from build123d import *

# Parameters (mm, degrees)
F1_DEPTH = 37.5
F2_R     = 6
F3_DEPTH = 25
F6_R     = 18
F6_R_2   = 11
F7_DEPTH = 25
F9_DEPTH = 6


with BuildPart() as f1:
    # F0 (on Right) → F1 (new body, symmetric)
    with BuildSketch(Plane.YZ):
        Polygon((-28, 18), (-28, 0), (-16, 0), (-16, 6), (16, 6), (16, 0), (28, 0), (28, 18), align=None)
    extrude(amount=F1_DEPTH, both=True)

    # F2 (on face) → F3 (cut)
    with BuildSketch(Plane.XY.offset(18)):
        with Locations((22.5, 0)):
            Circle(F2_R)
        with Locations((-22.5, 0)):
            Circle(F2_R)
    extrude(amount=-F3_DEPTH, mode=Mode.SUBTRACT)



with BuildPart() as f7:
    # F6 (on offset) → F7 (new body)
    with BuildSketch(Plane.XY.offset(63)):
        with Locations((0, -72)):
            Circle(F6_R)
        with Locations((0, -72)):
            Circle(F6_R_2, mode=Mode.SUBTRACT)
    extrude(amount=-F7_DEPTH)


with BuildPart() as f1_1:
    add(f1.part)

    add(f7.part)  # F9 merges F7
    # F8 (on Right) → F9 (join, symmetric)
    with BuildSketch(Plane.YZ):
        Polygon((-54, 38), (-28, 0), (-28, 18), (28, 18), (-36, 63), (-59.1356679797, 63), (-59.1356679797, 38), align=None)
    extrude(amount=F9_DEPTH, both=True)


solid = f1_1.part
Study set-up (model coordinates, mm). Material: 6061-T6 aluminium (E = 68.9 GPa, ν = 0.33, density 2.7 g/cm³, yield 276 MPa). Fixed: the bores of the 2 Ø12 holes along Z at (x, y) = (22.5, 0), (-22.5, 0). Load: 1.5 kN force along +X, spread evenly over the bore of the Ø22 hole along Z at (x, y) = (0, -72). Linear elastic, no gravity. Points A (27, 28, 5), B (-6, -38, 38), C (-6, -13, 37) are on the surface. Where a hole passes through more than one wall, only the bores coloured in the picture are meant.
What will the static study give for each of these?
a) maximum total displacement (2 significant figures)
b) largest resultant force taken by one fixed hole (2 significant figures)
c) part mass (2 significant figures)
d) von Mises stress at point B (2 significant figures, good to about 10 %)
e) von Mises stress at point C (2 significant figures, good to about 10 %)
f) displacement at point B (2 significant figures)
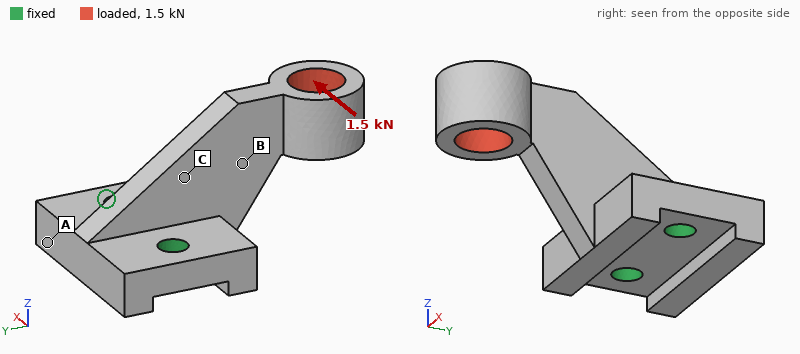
0.63 mm
2.7 kN
270 g
70 MPa
59 MPa
0.11 mm
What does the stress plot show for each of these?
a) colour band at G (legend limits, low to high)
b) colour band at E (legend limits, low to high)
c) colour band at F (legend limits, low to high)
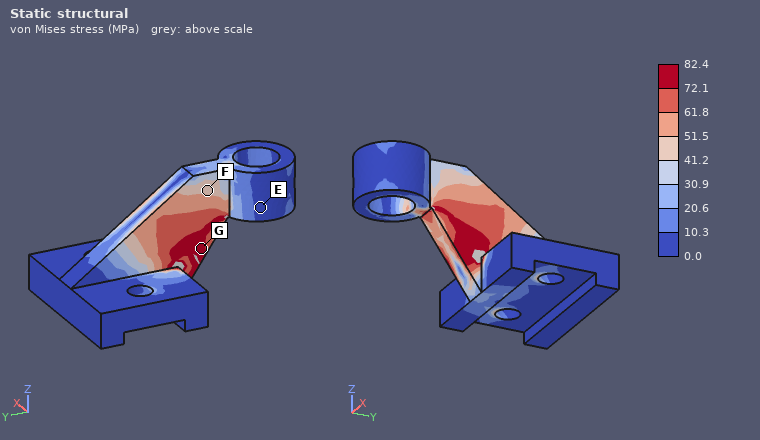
72.1 to 82.4 MPa
0.0 to 10.3 MPa
41.2 to 51.5 MPa
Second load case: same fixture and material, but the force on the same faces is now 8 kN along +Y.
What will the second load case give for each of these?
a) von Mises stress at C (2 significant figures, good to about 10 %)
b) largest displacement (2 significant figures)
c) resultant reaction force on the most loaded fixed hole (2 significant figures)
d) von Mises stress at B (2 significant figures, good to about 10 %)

47 MPa
0.45 mm
4.1 kN
28 MPa
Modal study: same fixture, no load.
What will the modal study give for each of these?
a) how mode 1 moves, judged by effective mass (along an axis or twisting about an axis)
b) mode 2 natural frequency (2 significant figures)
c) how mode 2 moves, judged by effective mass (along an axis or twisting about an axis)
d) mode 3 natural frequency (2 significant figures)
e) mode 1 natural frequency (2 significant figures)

along X
2100 Hz
along Z
3800 Hz
1300 Hz
